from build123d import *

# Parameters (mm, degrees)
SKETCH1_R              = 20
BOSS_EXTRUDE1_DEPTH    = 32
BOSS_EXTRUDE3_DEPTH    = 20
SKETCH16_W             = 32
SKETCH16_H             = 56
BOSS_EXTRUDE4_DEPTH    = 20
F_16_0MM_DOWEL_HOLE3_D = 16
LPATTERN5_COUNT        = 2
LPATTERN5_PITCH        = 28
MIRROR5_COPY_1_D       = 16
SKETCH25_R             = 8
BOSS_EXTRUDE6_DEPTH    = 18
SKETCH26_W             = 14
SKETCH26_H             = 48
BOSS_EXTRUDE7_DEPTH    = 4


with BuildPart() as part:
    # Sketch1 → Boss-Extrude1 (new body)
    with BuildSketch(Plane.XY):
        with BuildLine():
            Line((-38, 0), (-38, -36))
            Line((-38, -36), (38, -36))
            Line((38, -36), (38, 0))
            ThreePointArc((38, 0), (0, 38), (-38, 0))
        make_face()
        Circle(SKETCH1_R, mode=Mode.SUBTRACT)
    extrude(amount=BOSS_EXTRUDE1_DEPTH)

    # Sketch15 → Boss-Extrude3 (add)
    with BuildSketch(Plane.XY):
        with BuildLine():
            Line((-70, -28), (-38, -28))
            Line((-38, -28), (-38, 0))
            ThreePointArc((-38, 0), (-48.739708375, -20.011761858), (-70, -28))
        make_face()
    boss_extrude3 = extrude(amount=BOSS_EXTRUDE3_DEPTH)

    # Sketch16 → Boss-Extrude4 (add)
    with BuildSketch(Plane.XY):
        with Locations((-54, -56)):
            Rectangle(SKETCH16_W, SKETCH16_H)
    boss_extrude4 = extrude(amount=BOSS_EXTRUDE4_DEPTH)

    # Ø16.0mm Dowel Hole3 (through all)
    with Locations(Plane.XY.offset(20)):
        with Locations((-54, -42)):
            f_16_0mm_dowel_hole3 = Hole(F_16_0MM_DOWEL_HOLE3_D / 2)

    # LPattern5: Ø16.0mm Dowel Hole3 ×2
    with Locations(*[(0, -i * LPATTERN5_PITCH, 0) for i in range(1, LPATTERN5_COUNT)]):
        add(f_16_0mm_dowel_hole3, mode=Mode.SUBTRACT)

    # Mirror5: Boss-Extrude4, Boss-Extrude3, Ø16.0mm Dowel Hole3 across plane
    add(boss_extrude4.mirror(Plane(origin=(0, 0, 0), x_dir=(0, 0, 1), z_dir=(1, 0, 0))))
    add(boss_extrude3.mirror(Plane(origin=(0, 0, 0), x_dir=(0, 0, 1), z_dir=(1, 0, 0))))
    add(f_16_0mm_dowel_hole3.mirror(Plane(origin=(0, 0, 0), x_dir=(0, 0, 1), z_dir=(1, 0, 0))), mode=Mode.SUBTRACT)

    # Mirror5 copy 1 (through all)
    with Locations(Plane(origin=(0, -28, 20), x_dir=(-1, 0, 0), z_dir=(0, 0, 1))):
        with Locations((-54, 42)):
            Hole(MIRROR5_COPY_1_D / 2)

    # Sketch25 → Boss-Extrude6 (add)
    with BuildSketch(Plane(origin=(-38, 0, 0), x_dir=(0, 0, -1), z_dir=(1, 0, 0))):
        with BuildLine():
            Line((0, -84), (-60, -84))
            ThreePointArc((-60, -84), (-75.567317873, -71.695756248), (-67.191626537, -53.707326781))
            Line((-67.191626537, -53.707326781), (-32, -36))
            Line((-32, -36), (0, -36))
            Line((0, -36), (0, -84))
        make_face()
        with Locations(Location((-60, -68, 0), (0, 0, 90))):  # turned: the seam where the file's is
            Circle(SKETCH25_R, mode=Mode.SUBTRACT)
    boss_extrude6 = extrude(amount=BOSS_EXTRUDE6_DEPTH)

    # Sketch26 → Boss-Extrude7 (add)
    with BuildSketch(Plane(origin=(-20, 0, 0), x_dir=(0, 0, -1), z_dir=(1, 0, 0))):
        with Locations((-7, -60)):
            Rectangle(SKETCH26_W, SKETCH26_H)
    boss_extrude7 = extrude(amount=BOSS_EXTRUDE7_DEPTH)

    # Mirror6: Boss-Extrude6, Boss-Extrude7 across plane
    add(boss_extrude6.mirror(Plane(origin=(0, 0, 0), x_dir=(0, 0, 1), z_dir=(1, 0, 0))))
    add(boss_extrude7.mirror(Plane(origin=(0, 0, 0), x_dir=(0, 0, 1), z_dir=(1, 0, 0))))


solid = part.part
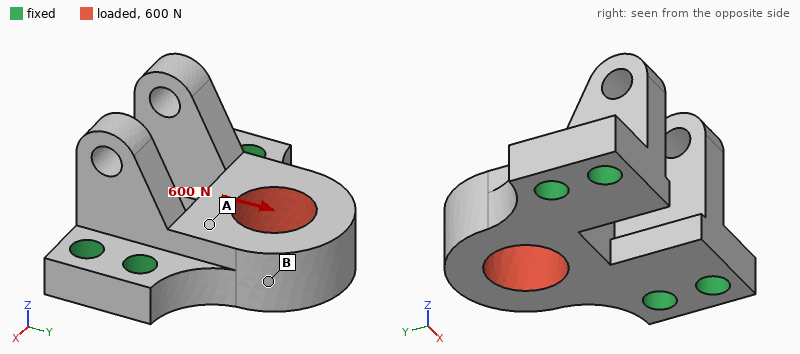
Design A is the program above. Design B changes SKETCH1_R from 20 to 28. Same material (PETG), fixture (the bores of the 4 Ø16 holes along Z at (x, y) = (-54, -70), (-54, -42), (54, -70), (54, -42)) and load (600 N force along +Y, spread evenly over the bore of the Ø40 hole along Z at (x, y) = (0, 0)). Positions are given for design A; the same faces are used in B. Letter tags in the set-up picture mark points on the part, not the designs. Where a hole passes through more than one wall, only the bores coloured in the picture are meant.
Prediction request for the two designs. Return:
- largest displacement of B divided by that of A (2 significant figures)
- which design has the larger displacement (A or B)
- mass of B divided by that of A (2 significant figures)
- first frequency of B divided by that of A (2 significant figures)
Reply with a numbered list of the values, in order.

1. 1.5
2. B
3. 0.87
4. 1.1
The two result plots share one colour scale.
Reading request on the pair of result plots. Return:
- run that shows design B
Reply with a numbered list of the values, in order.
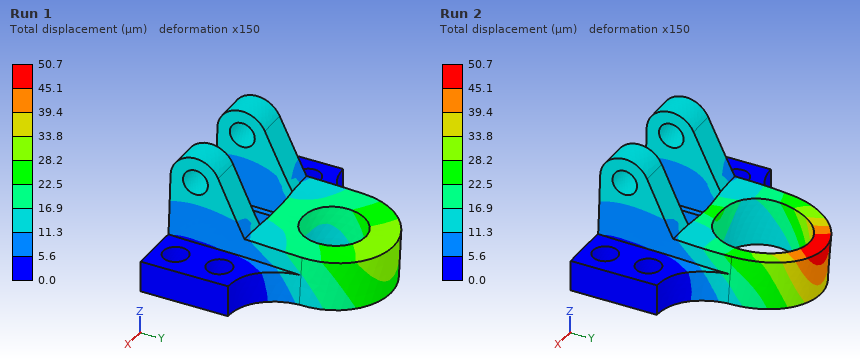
1. Run 2
